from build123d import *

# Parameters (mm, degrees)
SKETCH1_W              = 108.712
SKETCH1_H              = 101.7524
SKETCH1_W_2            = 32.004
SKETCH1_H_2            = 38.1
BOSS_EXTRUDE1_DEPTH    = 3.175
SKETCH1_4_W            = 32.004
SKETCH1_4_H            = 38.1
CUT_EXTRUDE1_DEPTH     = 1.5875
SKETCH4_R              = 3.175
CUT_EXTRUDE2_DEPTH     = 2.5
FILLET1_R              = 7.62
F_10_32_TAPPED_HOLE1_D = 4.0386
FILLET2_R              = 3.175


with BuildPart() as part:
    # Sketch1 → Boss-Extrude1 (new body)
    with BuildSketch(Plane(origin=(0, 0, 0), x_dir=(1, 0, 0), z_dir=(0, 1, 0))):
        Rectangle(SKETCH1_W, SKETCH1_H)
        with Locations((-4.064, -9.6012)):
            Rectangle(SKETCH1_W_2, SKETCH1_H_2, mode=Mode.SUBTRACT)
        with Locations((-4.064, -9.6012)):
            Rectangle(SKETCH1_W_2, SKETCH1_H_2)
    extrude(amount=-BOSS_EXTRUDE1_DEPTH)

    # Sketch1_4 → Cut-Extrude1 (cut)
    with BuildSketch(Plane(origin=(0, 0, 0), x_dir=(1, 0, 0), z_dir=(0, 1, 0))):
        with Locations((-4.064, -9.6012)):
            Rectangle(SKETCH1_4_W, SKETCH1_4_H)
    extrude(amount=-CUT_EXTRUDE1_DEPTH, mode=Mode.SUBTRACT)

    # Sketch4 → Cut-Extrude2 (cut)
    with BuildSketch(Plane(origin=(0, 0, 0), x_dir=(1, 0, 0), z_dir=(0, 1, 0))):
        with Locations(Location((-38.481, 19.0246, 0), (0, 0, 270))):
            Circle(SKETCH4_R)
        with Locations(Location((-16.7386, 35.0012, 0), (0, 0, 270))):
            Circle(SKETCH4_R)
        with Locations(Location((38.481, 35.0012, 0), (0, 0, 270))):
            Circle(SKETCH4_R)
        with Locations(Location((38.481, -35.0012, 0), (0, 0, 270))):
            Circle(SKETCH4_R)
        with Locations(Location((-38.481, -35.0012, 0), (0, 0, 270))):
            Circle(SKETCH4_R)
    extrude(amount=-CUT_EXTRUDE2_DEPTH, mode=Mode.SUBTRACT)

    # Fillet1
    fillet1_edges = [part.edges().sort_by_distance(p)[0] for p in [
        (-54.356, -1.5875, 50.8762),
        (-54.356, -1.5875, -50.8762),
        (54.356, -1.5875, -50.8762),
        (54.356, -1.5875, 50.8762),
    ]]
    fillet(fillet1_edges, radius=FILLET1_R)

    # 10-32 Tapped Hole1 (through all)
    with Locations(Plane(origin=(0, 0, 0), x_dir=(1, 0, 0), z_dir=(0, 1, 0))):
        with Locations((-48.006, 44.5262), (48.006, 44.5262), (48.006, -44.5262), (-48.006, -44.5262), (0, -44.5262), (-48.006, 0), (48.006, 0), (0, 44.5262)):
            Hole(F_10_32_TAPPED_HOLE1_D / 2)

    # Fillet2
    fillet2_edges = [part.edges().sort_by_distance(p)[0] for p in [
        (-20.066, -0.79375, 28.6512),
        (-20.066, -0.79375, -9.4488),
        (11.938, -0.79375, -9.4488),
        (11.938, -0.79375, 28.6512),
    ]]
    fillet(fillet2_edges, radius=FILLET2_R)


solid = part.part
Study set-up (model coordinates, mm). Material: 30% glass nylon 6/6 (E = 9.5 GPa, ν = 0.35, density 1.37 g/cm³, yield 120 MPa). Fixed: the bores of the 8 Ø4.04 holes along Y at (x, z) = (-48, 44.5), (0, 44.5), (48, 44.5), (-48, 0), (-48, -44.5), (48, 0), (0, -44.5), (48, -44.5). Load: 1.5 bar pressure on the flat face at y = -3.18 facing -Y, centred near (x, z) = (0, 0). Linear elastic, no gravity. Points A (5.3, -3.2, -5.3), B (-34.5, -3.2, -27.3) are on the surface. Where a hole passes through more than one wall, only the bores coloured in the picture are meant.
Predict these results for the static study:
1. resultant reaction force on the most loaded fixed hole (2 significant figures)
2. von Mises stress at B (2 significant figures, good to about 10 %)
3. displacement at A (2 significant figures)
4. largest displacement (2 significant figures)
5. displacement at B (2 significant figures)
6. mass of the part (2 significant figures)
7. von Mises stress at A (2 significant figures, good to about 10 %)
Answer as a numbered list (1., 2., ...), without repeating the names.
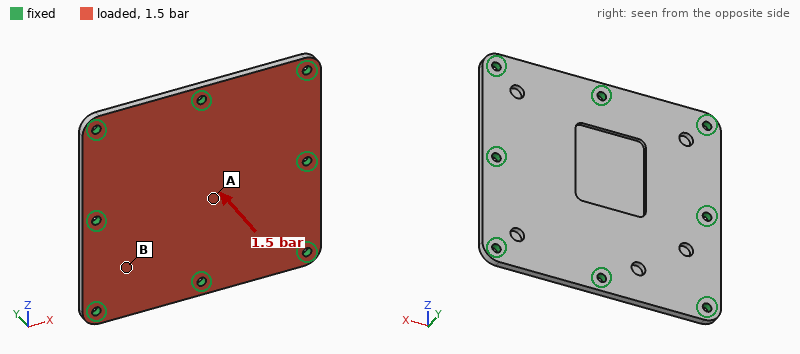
1. 360 N
2. 10 MPa
3. 0.85 mm
4. 0.95 mm
5. 0.21 mm
6. 44 g
7. 27 MPa
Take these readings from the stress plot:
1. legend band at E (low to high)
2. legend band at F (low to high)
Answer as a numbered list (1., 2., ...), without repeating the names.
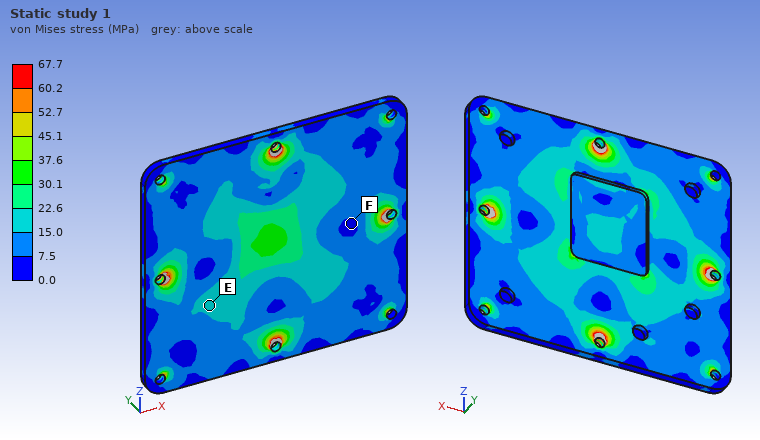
1. 15.0 to 22.6 MPa
2. 0.0 to 7.5 MPa
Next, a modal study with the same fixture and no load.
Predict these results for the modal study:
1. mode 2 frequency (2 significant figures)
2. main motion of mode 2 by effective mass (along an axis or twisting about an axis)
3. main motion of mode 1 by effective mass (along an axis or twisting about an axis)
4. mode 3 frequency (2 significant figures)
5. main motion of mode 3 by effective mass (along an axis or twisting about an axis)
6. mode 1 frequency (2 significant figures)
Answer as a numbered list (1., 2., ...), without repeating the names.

1. 2300 Hz
2. twisting about Z
3. along Y
4. 2600 Hz
5. twisting about X
6. 1500 Hz
